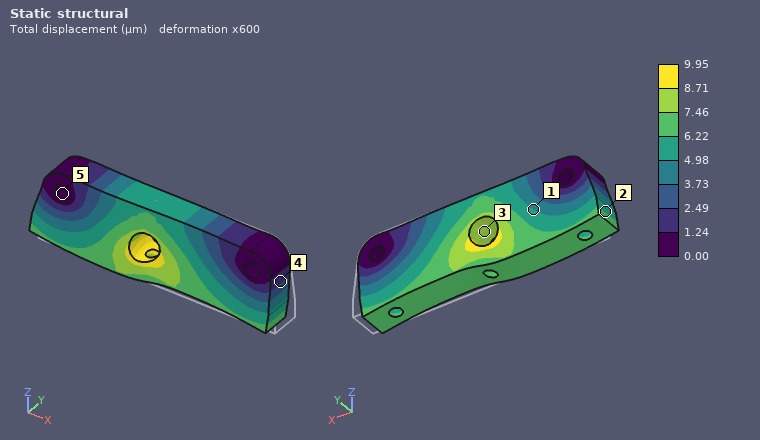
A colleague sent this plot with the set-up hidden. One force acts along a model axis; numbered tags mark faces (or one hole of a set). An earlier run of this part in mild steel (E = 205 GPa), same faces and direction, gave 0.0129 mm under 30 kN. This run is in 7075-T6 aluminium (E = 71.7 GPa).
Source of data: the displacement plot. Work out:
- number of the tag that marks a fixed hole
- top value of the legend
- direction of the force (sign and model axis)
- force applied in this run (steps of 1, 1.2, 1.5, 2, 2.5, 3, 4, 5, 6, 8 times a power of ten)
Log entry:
5
9.95 µm
-X
8 kN
